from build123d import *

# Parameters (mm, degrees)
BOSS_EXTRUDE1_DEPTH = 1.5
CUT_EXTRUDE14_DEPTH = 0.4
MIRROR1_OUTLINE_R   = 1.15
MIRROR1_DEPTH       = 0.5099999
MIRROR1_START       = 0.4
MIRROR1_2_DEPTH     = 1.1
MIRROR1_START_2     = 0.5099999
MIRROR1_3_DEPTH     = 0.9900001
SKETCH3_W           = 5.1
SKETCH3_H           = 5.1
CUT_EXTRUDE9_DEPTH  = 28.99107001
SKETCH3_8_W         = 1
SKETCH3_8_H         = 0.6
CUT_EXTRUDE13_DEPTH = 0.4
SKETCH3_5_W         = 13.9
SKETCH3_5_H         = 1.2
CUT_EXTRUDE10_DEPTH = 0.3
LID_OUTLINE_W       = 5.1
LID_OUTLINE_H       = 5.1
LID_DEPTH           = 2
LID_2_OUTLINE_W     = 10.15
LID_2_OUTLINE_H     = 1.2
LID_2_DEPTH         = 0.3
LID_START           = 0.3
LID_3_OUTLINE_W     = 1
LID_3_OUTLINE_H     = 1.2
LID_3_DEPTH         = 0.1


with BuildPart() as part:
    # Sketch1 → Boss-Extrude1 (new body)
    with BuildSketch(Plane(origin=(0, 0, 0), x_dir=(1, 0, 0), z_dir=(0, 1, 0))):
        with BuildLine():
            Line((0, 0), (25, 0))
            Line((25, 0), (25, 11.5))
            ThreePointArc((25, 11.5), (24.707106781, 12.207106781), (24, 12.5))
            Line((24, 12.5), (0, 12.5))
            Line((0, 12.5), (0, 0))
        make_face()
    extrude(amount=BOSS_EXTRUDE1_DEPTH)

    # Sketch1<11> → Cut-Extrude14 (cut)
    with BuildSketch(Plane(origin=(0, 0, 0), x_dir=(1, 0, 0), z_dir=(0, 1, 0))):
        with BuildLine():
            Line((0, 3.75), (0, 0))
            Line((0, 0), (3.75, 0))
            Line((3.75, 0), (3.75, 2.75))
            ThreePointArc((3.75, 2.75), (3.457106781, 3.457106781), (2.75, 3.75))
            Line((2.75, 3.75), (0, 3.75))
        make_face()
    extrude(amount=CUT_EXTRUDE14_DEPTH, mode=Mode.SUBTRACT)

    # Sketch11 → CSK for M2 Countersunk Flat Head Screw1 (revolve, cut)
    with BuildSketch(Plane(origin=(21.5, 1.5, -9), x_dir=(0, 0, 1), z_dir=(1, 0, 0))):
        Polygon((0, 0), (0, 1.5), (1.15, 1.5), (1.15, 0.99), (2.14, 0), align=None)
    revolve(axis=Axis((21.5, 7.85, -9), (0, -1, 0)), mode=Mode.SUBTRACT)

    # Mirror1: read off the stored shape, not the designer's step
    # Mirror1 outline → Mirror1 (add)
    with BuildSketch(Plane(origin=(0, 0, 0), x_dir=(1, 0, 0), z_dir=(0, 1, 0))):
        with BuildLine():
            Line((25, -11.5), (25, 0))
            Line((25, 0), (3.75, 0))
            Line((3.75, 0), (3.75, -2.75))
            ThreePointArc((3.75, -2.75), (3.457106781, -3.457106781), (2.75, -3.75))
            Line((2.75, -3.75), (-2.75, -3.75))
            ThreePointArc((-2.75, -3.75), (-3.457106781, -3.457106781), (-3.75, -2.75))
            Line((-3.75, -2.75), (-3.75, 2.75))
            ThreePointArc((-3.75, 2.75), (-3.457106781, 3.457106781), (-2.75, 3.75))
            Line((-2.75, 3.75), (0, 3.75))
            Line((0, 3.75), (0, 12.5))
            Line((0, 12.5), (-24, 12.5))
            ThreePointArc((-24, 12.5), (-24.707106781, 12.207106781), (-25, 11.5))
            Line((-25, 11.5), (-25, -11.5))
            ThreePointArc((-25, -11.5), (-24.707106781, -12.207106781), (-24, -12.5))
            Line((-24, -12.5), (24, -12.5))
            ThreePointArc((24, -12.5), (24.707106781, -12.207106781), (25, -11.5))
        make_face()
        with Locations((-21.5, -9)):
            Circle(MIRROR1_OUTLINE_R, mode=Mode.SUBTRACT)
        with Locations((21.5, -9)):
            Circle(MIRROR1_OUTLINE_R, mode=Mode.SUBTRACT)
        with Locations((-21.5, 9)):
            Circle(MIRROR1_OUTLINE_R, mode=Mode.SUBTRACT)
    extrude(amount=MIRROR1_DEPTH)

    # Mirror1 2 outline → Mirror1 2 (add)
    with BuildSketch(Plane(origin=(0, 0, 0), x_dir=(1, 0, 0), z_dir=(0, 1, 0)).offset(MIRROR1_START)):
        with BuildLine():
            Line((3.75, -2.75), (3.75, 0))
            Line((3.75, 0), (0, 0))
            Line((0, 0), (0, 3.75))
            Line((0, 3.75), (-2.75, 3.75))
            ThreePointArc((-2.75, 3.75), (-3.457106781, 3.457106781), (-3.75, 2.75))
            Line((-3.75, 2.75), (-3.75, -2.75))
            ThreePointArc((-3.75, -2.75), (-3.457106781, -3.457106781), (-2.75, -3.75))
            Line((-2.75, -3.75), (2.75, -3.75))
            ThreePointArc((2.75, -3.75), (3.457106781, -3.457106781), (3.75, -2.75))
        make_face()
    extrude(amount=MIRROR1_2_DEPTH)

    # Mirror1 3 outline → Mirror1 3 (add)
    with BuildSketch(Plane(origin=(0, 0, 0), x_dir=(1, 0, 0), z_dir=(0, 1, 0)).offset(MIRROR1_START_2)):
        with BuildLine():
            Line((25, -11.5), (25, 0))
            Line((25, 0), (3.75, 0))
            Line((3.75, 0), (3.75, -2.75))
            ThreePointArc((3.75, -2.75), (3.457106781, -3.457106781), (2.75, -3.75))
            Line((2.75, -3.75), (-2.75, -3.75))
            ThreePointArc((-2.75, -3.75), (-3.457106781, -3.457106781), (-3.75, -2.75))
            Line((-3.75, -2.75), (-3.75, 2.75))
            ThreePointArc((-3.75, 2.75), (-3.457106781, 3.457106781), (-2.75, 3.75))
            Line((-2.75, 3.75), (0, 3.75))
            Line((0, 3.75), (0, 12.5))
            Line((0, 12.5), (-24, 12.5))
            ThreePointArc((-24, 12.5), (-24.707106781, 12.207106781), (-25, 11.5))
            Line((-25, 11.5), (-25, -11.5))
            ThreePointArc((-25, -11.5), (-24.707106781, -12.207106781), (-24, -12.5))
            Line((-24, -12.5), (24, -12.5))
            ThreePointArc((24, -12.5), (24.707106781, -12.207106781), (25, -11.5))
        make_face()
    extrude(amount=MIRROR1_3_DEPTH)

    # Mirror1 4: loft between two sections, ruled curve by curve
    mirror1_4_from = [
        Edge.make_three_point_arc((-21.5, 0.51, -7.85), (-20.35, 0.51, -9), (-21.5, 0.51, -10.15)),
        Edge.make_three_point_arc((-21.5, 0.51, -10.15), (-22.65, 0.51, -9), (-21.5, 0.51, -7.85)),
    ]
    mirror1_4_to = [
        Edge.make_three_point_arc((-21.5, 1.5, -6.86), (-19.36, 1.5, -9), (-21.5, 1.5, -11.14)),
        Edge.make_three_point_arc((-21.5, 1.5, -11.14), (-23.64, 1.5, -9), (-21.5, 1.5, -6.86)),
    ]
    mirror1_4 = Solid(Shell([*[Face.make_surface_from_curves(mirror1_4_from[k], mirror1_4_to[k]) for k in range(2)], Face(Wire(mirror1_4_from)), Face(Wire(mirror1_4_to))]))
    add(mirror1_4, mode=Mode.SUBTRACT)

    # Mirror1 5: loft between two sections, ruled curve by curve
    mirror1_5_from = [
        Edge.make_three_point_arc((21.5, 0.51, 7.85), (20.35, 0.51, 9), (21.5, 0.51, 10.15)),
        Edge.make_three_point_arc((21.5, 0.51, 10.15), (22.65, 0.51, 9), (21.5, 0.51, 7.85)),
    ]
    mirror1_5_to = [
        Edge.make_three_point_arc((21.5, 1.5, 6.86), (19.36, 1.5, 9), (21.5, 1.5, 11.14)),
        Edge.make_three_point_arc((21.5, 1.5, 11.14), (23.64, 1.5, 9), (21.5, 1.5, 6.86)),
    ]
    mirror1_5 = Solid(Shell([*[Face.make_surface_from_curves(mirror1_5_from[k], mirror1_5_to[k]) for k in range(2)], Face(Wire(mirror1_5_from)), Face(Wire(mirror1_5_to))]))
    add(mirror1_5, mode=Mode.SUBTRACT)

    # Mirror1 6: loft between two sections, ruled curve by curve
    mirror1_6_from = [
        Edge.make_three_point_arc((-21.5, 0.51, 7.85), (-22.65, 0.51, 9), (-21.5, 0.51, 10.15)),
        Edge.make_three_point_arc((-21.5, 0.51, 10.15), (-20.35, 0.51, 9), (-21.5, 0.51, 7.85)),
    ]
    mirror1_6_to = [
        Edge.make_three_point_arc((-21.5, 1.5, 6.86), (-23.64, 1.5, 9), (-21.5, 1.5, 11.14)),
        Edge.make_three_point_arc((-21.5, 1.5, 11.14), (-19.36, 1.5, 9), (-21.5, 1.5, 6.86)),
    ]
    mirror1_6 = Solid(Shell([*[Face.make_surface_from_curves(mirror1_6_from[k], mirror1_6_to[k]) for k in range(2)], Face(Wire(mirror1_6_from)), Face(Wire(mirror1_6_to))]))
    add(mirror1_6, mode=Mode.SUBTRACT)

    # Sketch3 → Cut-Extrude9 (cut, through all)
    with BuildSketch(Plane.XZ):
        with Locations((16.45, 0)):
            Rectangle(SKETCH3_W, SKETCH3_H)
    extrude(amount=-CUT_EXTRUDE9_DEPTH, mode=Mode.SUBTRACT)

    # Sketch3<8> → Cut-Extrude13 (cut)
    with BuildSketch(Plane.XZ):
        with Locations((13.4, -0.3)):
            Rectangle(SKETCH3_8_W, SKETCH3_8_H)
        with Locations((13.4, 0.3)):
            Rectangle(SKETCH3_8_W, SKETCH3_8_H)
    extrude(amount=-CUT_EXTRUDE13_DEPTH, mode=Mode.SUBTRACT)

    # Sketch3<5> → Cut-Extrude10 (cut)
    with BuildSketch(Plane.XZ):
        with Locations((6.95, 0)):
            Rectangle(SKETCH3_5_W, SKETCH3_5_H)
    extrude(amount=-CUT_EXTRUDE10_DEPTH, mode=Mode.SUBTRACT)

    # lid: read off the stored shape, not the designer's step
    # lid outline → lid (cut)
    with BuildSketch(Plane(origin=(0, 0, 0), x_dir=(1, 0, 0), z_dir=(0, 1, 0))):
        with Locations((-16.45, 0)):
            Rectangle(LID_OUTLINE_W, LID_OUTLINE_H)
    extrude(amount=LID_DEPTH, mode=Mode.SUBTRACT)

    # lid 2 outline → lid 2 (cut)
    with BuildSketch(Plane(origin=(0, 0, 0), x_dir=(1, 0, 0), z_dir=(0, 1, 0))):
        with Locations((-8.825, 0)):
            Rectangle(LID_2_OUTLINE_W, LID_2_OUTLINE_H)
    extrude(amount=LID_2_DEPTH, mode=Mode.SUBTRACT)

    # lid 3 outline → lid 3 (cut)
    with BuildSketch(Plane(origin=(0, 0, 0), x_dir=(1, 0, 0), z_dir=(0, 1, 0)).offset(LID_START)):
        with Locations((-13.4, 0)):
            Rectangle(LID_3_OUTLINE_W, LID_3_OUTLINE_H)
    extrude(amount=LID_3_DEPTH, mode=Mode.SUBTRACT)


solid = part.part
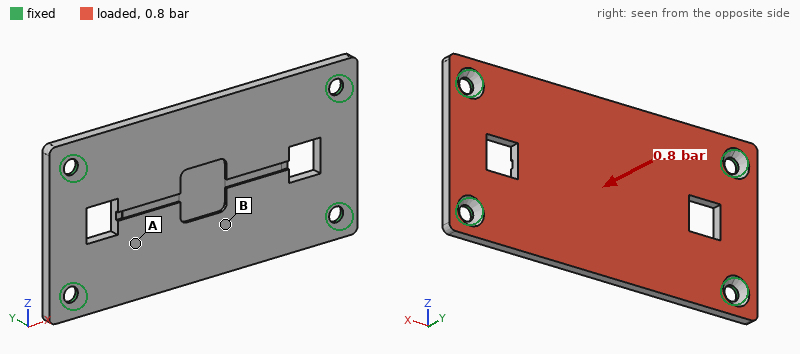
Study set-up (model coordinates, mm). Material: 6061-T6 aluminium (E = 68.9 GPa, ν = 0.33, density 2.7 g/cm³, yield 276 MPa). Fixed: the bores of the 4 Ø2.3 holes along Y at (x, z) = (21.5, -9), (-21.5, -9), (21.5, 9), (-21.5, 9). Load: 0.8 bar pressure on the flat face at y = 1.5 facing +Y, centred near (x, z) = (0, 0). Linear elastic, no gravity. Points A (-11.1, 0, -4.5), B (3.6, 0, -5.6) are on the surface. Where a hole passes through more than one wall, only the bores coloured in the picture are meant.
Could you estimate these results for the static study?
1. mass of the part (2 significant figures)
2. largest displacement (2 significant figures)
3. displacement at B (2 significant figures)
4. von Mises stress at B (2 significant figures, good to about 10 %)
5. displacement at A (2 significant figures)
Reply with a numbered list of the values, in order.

1. 4.7 g
2. 55 µm
3. 51 µm
4. 17 MPa
5. 32 µm
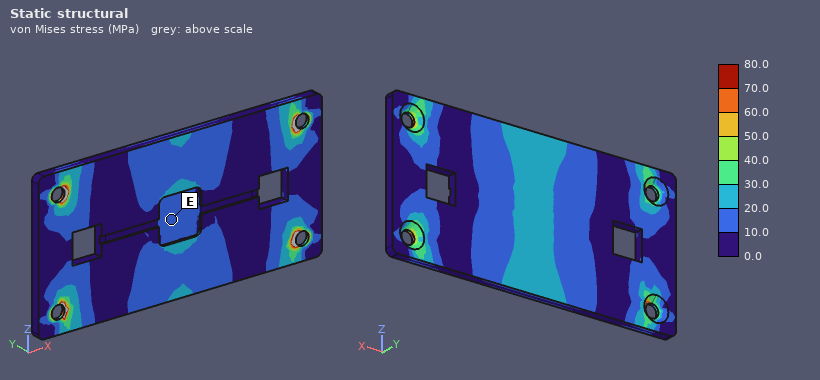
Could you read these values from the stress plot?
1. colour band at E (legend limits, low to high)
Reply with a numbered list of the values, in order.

1. 10.0 to 20.0 MPa
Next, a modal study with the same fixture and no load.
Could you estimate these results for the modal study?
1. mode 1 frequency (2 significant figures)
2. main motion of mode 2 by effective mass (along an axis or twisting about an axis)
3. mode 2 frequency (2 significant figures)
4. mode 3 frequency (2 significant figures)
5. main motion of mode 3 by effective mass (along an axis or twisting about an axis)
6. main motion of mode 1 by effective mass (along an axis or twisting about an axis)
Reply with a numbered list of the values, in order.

1. 3500 Hz
2. twisting about X
3. 5700 Hz
4. 9600 Hz
5. twisting about Z
6. along Y
